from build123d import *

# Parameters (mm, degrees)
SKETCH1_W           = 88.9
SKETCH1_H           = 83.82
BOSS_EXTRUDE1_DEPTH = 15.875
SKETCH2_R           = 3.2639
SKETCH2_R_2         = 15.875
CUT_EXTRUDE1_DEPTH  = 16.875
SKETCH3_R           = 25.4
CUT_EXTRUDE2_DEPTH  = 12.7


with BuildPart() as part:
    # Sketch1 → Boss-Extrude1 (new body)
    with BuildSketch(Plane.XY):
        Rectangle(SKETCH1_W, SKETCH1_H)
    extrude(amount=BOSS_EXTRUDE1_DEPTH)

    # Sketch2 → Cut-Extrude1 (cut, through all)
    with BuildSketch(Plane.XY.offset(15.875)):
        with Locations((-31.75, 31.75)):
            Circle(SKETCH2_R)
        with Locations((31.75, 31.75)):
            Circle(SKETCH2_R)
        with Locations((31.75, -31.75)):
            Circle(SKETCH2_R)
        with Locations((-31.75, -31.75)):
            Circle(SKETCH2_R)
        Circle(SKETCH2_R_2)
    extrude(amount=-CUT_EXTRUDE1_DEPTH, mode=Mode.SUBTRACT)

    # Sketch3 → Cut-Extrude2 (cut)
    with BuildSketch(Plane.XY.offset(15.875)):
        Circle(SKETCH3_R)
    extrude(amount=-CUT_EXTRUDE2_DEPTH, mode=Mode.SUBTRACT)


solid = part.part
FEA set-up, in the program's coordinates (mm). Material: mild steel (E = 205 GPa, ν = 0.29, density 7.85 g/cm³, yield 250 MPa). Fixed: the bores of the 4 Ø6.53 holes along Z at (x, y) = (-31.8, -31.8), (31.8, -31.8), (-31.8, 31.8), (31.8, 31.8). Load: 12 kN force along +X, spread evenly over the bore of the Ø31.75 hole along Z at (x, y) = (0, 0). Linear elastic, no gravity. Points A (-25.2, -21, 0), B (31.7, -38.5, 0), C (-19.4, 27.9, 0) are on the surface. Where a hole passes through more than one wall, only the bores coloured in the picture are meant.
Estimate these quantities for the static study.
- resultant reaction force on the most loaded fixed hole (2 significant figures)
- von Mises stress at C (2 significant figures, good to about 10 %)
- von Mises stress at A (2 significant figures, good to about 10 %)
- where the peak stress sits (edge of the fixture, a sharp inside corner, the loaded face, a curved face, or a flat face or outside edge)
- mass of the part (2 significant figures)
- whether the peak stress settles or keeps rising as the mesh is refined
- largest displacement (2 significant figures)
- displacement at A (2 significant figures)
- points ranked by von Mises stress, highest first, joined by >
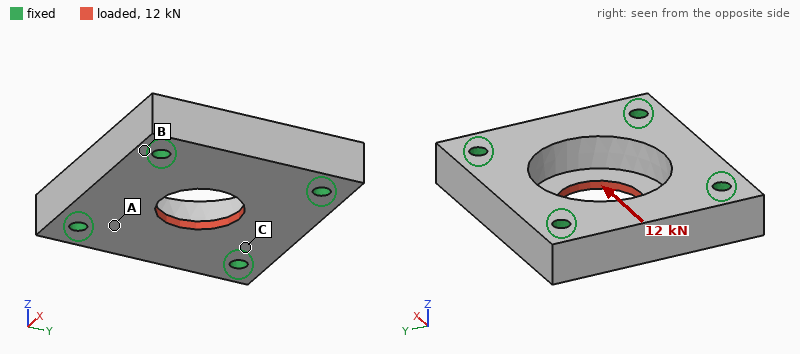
3.1 kN
14 MPa
24 MPa
a sharp inside corner
690 g
keeps rising
6.8 µm
1.5 µm
A > C > B
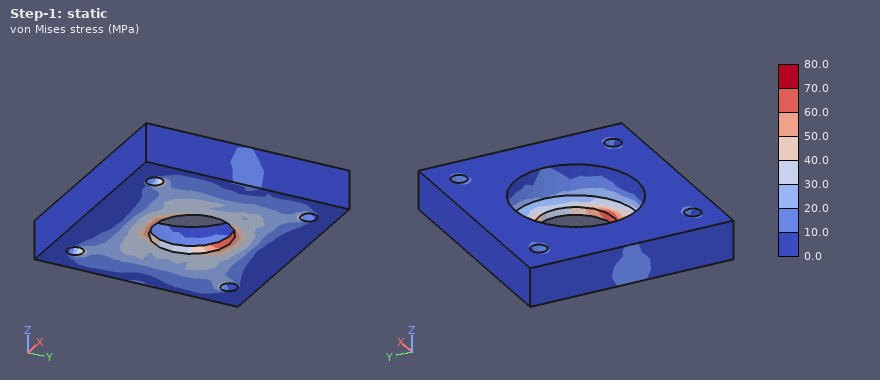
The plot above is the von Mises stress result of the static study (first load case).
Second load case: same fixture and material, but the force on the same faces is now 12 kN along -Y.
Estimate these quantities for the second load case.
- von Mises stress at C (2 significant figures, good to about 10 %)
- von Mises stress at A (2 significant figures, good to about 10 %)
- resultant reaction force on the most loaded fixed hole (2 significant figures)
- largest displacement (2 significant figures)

24 MPa
20 MPa
3.2 kN
7.0 µm
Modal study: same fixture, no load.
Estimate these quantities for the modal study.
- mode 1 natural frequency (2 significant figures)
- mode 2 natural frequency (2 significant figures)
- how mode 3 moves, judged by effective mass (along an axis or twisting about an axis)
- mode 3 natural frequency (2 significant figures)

14 kHz
14 kHz
twisting about Y
16 kHz
